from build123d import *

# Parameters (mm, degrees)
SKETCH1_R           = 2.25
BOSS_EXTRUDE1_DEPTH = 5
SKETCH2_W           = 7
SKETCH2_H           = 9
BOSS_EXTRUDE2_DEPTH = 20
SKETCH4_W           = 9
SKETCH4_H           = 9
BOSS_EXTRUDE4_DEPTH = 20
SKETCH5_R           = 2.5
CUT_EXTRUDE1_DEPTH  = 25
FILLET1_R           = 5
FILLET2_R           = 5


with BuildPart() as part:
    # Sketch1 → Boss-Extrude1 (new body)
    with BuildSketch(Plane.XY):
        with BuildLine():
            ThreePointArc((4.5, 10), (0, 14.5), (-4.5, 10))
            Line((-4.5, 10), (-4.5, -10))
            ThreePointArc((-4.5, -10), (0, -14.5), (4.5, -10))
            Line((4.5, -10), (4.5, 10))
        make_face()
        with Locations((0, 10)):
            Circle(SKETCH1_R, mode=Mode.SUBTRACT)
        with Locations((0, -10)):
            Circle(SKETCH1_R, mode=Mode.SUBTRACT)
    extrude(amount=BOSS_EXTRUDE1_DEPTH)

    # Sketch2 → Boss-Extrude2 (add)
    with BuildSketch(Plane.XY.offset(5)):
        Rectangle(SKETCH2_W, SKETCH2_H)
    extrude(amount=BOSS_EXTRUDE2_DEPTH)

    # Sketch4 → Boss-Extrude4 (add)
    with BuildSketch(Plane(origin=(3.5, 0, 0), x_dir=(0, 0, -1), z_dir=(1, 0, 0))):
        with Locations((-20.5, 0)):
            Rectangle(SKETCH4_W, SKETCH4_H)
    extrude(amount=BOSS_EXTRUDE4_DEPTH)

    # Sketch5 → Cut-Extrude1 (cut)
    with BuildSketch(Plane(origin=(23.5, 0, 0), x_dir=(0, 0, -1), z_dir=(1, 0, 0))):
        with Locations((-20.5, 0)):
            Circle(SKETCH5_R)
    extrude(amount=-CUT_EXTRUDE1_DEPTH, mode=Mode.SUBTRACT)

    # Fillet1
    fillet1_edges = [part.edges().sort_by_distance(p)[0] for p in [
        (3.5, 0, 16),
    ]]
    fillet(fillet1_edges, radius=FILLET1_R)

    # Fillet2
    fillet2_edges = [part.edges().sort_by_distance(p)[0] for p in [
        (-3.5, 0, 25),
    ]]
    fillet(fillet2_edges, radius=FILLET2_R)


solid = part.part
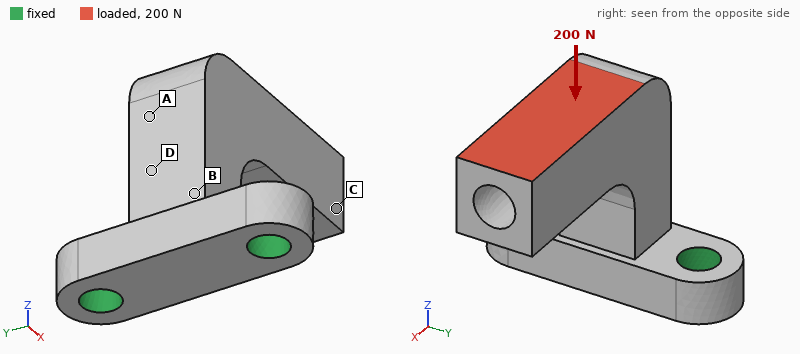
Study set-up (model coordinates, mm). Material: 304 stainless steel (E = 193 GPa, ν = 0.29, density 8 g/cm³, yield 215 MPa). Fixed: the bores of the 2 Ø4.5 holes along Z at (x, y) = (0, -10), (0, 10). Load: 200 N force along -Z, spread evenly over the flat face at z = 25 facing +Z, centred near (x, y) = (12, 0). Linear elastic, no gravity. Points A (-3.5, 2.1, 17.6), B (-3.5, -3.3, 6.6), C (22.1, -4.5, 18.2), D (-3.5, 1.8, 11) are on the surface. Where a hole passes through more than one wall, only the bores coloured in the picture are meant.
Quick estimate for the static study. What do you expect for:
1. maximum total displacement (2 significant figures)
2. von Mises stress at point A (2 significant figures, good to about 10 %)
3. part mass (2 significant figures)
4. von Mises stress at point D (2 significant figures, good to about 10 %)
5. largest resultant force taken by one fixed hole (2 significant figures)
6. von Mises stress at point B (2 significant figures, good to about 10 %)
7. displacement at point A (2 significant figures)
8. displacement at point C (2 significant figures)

31 µm
15 MPa
28 g
29 MPa
100 N
33 MPa
9.8 µm
26 µm
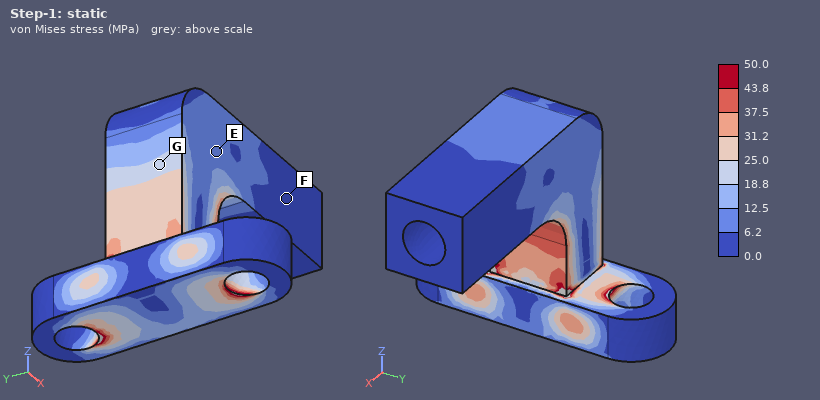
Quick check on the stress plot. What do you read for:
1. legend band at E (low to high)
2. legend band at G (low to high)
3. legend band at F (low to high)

6.2 to 12.5 MPa
18.8 to 25.0 MPa
0.0 to 6.2 MPa
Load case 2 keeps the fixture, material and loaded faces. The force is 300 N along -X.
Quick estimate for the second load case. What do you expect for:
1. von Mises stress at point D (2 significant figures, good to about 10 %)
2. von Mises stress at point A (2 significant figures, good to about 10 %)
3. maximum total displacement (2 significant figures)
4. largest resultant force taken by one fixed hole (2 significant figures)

55 MPa
21 MPa
64 µm
150 N
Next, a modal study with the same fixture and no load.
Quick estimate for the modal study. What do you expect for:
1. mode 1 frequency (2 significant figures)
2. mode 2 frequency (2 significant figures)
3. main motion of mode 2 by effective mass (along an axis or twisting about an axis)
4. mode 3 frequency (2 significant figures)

3700 Hz
4900 Hz
along Y
12 kHz
